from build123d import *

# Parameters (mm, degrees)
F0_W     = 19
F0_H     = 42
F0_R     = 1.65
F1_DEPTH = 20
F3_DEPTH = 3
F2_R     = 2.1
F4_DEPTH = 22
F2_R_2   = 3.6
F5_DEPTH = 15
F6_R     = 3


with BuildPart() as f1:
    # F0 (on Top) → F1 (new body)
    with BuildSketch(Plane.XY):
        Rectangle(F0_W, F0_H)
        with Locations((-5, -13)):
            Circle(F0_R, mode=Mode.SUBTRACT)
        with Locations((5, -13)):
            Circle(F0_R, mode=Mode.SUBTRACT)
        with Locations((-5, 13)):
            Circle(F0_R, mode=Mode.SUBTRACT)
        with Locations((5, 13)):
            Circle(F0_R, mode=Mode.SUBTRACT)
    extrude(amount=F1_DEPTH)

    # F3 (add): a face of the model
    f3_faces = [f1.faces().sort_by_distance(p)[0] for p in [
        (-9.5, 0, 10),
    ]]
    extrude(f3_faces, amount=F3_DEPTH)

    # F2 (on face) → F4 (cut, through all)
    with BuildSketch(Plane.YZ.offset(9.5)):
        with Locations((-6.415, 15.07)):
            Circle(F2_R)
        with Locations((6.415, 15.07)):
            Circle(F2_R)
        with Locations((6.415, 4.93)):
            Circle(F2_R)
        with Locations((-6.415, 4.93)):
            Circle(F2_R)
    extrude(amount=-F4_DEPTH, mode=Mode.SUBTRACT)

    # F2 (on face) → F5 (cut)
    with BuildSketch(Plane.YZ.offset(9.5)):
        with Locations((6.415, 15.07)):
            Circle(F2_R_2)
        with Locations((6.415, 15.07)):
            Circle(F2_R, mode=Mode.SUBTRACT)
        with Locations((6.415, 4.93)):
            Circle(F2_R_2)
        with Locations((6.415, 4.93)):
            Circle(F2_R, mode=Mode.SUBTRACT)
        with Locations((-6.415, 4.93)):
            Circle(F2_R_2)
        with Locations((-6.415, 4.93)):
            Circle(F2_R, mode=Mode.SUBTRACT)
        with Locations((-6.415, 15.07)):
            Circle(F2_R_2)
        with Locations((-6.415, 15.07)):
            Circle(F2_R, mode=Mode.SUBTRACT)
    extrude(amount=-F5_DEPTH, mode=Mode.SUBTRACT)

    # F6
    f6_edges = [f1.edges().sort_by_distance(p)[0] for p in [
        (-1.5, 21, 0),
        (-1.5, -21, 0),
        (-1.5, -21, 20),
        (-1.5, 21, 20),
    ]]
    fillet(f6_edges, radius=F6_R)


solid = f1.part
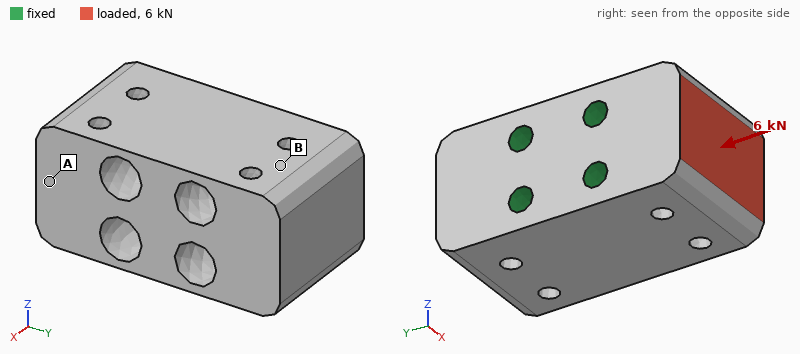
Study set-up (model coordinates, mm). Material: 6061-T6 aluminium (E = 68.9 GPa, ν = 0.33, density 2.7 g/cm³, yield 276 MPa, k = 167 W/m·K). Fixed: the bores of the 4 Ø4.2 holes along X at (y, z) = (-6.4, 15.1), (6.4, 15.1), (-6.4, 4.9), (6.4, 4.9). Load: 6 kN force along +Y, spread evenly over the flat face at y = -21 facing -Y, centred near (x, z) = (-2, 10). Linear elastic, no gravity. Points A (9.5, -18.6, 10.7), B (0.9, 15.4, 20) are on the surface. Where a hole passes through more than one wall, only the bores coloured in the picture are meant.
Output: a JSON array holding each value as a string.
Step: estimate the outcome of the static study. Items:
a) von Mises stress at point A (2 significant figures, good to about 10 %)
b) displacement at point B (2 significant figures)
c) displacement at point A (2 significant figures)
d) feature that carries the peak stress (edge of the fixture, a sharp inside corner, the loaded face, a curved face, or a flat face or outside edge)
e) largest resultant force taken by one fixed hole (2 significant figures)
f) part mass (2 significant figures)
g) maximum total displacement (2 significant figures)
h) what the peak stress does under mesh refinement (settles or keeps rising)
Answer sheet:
["21 MPa", "7.7 µm", "23 µm", "edge of the fixture", "2.3 kN", "40 g", "25 µm", "keeps rising"]
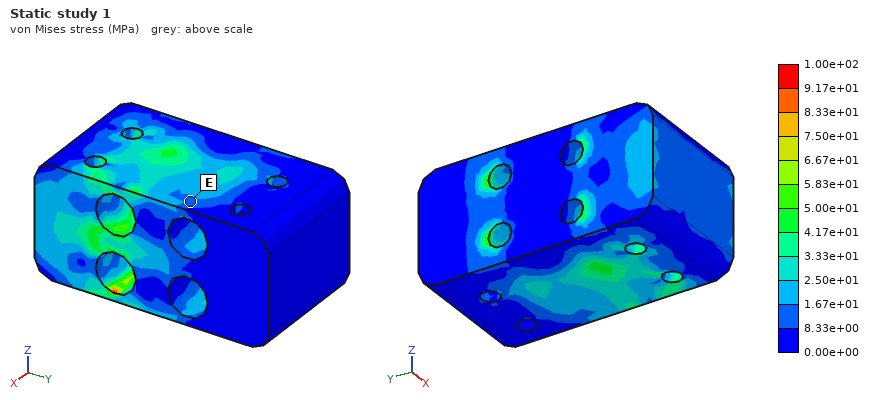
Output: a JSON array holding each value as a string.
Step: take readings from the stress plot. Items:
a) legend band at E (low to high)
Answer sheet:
["8.33e+00 to 1.67e+01 MPa"]
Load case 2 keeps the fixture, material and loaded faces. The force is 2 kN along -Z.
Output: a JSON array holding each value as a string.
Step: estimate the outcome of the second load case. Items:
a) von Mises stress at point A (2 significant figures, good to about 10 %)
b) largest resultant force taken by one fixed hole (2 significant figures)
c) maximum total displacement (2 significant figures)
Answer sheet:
["9.4 MPa", "2.0 kN", "17 µm"]
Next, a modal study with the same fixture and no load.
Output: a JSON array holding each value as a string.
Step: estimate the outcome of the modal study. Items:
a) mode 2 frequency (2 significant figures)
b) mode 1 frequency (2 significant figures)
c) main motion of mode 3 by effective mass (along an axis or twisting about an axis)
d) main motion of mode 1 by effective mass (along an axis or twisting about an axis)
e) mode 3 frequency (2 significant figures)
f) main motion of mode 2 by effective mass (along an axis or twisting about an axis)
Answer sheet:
["19 kHz", "16 kHz", "twisting about X", "along Y", "21 kHz", "along Z"]
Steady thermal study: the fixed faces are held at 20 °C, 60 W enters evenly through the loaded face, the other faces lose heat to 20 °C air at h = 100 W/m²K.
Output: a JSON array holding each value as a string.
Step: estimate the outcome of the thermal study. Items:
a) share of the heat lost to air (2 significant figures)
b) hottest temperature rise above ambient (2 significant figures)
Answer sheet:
["5.3 %", "22 K"]
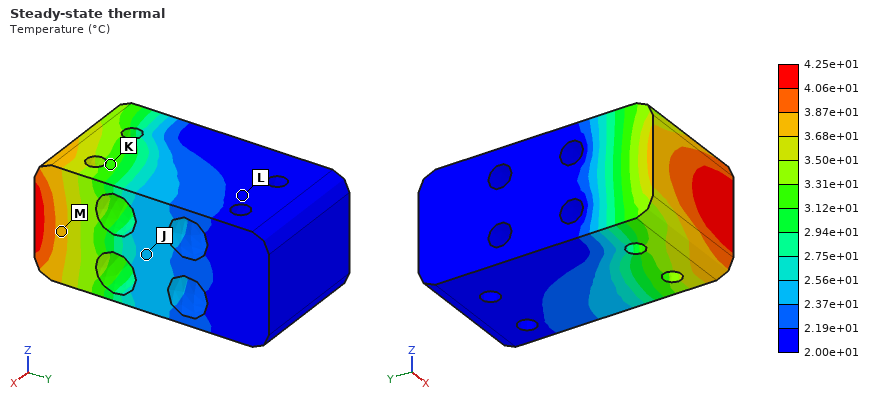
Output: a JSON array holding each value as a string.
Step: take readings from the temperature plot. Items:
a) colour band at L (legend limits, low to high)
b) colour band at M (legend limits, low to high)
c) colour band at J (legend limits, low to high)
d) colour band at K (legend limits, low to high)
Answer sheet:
["2.00e+01 to 2.19e+01 °C", "3.68e+01 to 3.87e+01 °C", "2.37e+01 to 2.56e+01 °C", "3.12e+01 to 3.31e+01 °C"]
